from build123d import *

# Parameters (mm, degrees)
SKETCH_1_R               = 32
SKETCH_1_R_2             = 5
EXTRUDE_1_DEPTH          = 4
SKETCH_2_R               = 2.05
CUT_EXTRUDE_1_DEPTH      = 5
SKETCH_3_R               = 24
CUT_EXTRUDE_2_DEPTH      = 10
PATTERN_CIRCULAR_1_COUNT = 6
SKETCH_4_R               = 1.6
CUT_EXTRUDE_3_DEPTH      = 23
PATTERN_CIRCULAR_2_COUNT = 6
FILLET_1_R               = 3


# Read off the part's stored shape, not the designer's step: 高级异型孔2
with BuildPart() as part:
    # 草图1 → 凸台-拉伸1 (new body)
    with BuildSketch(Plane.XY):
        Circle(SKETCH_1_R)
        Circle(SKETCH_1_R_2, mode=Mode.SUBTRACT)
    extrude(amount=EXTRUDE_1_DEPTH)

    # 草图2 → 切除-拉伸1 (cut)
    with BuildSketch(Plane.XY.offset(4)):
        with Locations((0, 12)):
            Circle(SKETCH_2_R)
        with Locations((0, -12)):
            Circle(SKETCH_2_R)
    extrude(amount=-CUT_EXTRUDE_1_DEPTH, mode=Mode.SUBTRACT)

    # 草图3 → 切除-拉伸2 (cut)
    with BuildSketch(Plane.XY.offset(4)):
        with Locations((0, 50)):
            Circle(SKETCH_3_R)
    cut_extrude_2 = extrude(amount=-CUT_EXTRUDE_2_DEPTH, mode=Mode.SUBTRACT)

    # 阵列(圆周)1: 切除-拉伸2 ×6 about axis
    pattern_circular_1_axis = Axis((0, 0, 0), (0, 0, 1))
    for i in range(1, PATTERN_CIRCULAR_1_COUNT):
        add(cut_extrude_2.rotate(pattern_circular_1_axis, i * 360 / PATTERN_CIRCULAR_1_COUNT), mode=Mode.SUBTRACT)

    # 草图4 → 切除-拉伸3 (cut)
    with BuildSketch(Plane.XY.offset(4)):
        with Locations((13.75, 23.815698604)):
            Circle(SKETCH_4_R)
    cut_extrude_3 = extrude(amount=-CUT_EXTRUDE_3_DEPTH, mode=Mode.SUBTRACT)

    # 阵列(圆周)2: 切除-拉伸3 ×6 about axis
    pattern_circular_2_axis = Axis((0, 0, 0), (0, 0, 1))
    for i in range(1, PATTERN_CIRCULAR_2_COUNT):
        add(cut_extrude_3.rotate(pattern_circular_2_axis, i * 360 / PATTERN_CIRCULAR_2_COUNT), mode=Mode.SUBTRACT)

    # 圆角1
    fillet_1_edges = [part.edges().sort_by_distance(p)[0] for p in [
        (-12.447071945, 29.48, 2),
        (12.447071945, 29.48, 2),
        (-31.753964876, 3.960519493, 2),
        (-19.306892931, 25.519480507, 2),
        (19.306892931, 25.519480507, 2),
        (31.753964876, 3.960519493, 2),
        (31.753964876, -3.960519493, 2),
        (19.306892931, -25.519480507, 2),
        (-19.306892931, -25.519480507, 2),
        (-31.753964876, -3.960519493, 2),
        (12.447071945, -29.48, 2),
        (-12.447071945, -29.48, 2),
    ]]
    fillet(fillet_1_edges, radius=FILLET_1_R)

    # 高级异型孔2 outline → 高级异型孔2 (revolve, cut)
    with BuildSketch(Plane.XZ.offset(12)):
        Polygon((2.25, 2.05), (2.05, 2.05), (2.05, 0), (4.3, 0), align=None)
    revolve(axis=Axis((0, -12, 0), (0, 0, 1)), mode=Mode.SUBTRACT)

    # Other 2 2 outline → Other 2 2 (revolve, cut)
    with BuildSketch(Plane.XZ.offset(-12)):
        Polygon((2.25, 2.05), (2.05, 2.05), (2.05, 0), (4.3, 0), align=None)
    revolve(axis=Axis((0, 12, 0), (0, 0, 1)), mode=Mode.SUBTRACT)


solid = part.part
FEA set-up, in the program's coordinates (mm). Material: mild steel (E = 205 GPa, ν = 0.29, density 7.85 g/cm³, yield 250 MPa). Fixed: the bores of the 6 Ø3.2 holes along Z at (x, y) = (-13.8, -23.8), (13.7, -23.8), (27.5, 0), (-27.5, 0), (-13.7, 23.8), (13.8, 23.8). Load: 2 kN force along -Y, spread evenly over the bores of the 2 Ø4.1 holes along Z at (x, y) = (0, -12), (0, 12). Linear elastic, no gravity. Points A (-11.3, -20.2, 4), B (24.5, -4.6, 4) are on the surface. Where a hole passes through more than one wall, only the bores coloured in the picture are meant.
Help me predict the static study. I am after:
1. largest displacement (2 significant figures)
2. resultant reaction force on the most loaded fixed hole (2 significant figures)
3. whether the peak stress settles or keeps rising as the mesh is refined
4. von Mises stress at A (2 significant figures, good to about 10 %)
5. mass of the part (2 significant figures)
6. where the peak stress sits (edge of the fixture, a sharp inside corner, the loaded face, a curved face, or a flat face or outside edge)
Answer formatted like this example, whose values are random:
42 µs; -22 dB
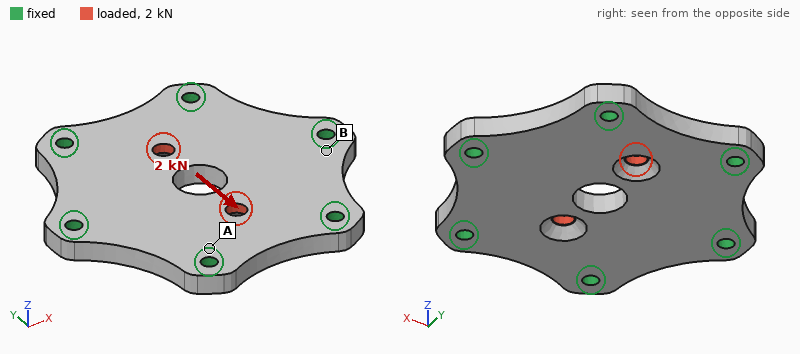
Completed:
1.9 µm; 480 N; keeps rising; 16 MPa; 76 g; a sharp inside corner
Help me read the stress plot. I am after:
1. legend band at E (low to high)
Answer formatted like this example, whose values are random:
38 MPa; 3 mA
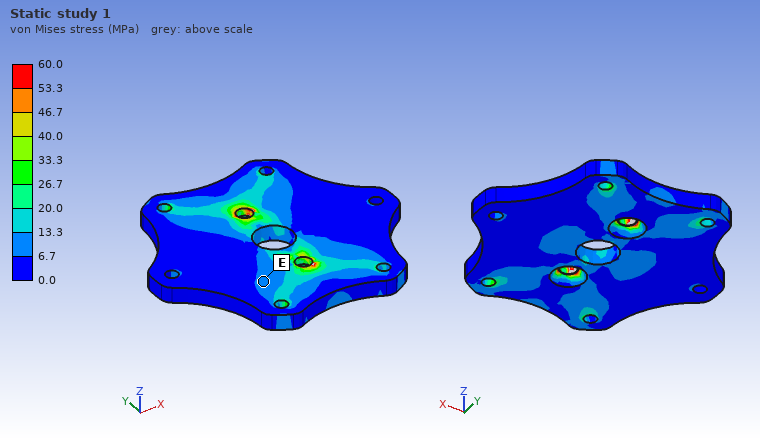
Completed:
6.7 to 13.3 MPa
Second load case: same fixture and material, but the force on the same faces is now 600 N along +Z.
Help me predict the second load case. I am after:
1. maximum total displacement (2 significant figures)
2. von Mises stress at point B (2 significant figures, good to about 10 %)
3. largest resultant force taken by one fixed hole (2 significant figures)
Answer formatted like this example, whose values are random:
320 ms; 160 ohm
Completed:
7.7 µm; 12 MPa; 130 N
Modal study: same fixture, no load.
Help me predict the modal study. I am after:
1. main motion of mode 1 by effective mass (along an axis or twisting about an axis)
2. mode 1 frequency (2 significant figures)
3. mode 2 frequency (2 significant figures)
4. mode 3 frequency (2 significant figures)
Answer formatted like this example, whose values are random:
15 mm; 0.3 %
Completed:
along Z; 10 kHz; 20 kHz; 20 kHz
